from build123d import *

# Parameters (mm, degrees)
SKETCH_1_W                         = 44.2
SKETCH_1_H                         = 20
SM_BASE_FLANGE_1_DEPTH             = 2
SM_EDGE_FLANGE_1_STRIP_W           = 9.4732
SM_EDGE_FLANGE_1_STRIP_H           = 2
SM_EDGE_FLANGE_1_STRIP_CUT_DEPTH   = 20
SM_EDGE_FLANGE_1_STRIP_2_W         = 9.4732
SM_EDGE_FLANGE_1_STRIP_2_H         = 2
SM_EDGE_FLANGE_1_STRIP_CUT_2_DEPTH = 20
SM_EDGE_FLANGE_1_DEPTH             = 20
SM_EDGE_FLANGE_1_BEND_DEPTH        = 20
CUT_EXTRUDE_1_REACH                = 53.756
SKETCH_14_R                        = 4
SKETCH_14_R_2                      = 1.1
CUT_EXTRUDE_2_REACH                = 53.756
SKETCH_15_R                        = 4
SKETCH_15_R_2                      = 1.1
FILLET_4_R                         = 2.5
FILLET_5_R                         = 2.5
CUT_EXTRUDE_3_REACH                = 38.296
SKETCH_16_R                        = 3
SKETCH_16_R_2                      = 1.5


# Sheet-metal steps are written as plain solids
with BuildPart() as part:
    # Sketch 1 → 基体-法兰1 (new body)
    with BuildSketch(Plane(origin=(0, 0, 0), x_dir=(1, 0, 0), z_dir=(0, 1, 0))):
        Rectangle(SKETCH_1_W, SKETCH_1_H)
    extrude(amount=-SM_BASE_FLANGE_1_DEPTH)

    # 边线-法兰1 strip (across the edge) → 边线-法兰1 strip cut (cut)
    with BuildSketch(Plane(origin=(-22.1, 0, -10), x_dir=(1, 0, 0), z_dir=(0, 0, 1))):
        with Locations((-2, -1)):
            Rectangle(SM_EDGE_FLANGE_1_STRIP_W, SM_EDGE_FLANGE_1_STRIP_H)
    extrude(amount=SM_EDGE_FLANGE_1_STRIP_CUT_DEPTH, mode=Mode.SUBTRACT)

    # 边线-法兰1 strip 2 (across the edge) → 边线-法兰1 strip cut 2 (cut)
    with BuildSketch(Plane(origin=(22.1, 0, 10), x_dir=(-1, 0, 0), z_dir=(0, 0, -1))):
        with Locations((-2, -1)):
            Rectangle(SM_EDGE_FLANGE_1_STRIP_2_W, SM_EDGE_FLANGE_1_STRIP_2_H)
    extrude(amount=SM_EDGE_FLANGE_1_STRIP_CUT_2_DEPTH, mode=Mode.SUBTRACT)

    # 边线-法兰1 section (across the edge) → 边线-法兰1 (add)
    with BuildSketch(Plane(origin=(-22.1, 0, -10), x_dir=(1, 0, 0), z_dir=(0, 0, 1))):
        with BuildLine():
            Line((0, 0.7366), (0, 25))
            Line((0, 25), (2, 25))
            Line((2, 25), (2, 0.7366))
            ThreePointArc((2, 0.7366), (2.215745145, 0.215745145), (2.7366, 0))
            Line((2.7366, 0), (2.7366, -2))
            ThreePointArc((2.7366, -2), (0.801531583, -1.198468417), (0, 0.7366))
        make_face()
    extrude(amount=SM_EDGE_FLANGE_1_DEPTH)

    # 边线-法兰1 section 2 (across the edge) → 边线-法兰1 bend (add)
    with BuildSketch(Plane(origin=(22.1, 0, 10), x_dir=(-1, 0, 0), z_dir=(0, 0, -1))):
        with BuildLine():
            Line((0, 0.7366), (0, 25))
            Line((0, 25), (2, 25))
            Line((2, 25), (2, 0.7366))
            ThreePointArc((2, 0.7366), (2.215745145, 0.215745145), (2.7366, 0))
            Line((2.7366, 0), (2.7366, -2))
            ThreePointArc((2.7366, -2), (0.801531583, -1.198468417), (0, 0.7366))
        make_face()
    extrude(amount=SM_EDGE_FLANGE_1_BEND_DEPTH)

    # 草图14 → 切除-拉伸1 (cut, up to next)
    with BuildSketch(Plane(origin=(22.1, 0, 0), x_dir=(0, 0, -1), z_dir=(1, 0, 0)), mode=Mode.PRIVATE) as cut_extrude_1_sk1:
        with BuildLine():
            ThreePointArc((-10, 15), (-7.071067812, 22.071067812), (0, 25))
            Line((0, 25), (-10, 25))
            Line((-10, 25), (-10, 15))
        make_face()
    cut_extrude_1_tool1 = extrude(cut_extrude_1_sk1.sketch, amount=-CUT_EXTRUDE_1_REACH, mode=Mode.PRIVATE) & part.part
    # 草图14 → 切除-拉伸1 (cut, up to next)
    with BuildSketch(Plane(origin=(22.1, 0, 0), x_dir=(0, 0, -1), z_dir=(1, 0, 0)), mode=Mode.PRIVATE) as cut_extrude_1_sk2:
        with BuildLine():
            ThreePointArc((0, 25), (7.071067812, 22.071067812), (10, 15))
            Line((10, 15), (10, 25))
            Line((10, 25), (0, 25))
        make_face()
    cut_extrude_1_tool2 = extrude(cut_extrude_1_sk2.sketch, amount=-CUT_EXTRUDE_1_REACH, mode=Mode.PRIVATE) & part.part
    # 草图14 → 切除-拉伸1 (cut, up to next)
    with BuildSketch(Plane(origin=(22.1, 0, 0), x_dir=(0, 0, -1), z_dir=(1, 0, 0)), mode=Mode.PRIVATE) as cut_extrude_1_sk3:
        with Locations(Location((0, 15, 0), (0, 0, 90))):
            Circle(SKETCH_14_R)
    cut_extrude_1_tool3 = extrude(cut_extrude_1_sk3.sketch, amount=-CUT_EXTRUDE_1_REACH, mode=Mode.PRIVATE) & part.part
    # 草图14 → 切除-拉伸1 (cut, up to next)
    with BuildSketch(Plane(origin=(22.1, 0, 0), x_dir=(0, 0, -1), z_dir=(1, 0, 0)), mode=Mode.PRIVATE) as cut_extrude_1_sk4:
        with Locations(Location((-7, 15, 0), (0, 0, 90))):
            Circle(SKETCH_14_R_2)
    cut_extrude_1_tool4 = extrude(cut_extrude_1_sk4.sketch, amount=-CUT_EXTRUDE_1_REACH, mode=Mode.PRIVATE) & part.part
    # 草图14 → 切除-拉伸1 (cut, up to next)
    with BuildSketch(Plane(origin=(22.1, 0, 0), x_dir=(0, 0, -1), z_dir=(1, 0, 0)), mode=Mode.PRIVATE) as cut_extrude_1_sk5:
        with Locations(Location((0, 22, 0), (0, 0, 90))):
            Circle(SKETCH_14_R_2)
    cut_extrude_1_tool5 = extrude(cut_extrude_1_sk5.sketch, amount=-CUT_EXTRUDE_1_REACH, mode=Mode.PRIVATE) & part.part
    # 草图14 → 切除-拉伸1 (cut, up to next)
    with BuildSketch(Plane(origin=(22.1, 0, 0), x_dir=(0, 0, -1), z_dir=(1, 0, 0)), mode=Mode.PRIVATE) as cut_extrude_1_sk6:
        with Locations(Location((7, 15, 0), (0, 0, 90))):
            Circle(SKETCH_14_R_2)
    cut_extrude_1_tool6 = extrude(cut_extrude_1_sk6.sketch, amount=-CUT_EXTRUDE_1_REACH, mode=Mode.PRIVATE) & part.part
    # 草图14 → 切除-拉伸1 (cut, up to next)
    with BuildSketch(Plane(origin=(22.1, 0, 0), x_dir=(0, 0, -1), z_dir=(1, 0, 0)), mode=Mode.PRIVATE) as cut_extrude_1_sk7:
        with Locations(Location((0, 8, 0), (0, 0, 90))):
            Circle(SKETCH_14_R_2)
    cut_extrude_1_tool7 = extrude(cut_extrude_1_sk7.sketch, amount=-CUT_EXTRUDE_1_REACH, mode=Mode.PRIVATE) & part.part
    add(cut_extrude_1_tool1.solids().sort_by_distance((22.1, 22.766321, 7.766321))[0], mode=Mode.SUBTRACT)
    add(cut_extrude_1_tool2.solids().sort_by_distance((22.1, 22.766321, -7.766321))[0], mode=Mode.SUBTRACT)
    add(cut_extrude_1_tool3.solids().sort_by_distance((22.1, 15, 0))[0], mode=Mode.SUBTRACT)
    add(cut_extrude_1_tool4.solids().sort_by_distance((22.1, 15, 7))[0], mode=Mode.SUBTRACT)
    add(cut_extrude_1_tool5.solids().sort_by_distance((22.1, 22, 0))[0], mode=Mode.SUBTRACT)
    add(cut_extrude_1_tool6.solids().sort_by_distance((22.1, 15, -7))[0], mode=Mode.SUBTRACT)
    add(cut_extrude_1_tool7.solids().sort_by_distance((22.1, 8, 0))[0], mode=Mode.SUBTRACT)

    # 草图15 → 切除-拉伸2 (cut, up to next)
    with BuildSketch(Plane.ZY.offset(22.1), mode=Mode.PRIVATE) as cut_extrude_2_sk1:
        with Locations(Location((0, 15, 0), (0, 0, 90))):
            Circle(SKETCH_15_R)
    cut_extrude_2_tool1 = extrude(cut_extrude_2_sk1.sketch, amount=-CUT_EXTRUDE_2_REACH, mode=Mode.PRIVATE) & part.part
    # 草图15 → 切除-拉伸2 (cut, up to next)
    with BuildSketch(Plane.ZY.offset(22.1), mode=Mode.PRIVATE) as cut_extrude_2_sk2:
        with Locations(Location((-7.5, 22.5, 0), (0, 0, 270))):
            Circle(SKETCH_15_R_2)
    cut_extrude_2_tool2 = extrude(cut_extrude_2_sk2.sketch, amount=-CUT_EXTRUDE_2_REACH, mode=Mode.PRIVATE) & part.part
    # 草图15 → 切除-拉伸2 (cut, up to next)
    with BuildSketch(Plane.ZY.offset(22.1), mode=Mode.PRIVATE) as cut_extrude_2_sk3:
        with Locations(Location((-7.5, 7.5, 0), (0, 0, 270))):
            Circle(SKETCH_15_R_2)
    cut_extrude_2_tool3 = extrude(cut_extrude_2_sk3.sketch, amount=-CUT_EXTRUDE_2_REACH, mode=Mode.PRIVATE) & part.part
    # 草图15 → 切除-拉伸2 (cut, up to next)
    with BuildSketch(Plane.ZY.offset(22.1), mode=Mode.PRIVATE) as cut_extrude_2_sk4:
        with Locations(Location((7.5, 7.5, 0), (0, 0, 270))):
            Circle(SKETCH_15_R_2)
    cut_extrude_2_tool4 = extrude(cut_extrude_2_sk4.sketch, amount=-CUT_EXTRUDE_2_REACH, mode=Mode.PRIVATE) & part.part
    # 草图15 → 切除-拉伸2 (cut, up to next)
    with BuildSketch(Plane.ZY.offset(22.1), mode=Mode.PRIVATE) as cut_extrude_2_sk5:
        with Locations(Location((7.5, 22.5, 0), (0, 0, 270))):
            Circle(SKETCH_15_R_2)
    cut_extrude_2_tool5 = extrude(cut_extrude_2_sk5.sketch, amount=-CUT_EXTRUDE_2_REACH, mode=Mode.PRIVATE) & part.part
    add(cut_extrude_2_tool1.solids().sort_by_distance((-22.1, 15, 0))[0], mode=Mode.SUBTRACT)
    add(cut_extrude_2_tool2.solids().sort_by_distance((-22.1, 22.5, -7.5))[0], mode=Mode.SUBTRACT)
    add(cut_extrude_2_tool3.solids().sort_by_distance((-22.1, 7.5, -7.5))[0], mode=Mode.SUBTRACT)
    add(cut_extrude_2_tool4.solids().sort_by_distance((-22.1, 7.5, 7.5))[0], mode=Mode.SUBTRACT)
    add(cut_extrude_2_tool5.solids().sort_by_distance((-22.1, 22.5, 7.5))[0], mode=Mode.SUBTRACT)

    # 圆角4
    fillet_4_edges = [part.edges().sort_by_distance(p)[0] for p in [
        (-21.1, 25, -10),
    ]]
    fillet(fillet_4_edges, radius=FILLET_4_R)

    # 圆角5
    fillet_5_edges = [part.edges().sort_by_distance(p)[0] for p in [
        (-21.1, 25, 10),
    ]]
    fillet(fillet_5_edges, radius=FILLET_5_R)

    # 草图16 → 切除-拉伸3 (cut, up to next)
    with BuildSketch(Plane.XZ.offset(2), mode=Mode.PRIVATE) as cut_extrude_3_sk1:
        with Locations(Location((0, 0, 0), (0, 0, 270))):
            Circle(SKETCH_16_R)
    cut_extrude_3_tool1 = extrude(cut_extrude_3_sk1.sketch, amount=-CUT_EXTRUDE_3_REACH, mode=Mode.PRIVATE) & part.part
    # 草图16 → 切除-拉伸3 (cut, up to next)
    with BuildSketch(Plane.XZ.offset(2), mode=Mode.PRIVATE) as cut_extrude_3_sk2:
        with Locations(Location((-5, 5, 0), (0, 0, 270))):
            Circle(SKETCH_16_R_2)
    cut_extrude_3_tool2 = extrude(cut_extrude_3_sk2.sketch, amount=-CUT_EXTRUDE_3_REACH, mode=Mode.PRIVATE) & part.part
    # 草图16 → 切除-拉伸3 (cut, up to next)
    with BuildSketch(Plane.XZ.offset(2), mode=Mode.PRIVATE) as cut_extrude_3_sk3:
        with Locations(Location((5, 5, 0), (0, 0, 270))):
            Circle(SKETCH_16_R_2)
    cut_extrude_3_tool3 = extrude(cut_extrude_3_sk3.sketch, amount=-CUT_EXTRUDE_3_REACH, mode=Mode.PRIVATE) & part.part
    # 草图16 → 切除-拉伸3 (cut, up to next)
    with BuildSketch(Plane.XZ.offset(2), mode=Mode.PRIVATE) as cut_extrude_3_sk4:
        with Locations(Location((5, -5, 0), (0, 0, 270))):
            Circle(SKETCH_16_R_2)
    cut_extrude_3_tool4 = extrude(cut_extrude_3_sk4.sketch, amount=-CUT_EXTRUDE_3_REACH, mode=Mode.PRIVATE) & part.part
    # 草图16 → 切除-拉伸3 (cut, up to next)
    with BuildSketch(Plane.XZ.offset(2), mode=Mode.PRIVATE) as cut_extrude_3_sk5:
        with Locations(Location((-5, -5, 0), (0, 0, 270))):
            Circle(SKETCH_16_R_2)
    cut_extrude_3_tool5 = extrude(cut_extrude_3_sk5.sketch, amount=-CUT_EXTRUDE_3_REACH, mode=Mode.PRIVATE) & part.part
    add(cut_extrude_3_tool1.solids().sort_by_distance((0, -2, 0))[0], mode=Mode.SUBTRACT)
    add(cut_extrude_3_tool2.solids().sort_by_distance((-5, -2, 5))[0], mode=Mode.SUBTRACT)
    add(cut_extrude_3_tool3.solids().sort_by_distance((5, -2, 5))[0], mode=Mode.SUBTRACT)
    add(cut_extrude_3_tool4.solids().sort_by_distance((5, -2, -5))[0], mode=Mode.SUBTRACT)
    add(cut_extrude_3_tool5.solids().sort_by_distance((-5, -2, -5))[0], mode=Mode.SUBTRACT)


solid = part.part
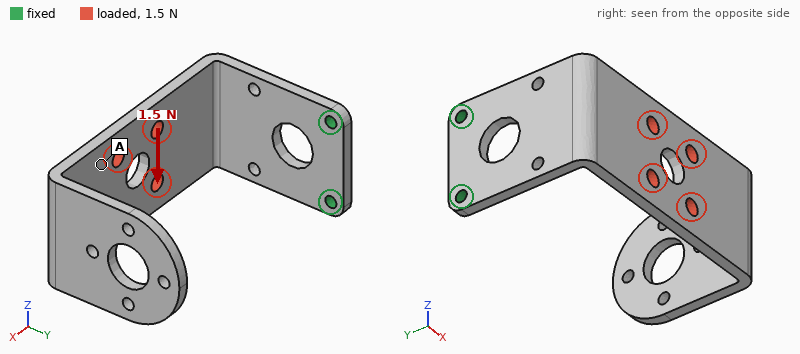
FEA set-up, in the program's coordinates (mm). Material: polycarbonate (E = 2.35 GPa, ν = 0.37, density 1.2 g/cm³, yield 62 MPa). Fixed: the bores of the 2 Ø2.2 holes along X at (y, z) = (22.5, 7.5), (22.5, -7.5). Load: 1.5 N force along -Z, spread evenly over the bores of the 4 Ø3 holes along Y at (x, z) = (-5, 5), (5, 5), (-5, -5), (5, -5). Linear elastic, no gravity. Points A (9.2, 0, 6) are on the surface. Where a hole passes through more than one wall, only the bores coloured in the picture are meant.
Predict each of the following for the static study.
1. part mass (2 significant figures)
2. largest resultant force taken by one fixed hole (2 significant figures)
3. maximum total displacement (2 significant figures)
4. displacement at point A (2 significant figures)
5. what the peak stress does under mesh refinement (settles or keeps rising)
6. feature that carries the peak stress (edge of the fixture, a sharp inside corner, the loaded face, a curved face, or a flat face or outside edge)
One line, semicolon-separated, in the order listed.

3.9 g; 3.0 N; 0.65 mm; 0.43 mm; keeps rising; edge of the fixture
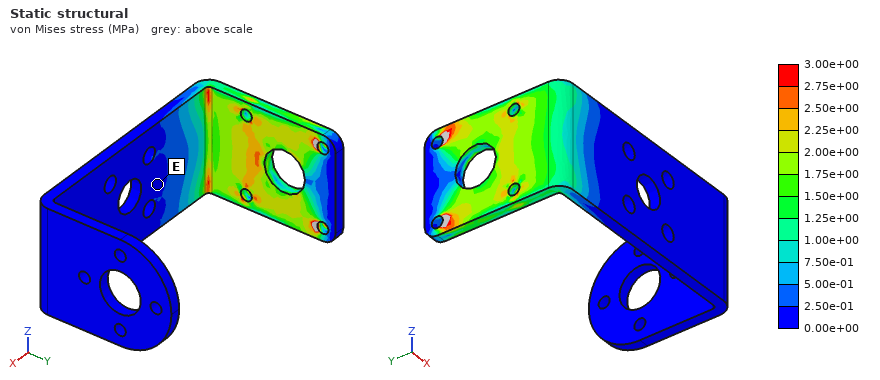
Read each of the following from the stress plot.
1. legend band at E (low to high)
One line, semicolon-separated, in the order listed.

0.00e+00 to 2.50e-01 MPa
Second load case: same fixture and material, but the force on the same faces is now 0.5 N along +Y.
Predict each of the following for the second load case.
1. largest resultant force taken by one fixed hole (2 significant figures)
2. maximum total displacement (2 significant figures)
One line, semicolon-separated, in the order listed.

0.25 N; 0.59 mm
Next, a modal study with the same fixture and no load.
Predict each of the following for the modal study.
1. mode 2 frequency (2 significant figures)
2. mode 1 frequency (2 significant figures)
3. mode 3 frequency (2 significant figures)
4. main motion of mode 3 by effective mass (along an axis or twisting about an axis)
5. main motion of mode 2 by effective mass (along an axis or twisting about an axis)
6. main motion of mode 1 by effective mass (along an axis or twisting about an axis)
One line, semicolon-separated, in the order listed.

130 Hz; 78 Hz; 260 Hz; along X; along Z; along Y
